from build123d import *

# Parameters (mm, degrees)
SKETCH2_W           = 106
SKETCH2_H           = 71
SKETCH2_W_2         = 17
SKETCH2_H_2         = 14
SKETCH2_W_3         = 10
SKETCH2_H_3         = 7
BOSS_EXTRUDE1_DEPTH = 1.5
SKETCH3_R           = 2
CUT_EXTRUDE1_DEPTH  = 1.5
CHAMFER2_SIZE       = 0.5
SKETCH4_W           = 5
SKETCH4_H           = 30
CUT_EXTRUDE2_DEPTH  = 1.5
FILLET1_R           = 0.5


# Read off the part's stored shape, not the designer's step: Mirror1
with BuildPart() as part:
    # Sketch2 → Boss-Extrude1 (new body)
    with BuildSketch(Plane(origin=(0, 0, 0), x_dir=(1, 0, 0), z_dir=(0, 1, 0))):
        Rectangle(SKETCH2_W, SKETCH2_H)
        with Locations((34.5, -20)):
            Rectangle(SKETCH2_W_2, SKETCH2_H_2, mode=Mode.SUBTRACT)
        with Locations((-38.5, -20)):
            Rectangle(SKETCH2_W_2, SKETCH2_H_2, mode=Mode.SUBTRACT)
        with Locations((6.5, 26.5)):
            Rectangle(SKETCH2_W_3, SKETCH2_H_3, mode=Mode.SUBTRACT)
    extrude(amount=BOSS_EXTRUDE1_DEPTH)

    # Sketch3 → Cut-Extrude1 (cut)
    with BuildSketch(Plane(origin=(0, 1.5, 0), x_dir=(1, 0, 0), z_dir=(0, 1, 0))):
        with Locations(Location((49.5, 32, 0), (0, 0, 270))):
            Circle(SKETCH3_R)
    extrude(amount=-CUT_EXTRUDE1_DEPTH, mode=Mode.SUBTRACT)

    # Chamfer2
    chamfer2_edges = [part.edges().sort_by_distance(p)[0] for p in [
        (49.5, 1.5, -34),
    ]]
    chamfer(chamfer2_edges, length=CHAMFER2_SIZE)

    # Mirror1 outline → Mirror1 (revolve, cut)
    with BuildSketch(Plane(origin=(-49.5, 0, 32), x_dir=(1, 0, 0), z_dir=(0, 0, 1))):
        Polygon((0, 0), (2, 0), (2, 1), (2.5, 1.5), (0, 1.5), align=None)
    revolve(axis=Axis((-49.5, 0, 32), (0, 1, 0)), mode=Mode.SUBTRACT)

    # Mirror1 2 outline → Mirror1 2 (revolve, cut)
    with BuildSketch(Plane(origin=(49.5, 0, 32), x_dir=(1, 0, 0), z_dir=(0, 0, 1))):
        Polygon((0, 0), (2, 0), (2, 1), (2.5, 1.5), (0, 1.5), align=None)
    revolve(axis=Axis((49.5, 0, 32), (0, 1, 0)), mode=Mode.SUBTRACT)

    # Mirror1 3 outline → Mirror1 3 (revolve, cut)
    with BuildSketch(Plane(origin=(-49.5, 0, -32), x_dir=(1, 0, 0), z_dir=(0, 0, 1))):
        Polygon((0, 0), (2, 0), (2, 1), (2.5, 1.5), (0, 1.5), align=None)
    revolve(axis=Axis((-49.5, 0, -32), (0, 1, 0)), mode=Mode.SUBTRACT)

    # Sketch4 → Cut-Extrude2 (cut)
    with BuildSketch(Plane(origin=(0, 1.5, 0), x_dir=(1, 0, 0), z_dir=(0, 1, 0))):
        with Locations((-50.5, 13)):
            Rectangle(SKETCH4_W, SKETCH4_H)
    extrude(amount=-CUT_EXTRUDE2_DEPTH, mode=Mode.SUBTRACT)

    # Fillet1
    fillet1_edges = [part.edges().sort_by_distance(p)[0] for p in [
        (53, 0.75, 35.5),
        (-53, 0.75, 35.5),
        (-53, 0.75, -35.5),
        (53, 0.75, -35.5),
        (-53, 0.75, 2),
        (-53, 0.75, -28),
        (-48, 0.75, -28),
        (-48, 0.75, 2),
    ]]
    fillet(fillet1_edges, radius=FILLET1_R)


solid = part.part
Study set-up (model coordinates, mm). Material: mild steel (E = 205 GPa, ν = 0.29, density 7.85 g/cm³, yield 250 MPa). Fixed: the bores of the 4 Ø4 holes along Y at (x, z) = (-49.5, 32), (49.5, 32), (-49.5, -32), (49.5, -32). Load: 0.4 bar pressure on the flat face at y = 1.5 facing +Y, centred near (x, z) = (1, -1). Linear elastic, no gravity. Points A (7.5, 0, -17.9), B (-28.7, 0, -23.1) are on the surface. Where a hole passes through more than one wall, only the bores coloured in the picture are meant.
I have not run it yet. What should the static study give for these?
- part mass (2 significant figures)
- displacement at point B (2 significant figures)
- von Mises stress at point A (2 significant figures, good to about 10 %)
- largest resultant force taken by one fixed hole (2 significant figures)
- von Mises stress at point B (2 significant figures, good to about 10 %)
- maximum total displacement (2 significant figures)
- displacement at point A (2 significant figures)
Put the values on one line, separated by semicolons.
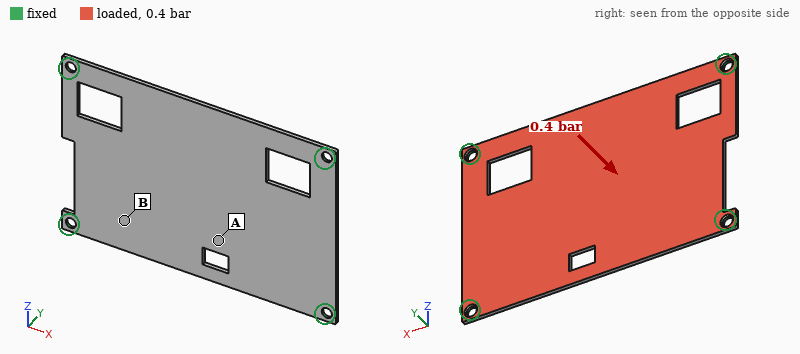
80 g; 0.16 mm; 59 MPa; 80 N; 22 MPa; 0.31 mm; 0.29 mm
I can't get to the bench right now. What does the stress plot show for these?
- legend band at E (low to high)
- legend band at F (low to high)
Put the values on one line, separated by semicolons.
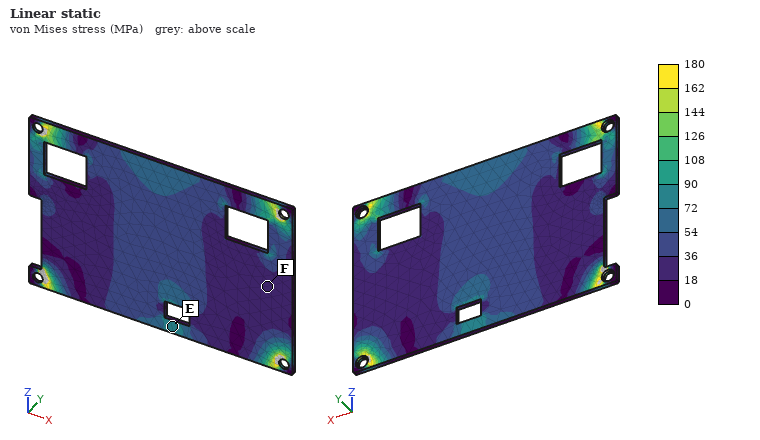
72 to 90 MPa; 18 to 36 MPa
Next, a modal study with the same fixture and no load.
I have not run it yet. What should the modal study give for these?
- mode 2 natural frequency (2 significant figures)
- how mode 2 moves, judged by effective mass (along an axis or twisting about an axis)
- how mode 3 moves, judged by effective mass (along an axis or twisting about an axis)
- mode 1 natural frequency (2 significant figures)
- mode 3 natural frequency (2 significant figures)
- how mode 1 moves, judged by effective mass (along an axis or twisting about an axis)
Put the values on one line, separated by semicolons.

1000 Hz; twisting about X; twisting about Z; 600 Hz; 1500 Hz; along Y
